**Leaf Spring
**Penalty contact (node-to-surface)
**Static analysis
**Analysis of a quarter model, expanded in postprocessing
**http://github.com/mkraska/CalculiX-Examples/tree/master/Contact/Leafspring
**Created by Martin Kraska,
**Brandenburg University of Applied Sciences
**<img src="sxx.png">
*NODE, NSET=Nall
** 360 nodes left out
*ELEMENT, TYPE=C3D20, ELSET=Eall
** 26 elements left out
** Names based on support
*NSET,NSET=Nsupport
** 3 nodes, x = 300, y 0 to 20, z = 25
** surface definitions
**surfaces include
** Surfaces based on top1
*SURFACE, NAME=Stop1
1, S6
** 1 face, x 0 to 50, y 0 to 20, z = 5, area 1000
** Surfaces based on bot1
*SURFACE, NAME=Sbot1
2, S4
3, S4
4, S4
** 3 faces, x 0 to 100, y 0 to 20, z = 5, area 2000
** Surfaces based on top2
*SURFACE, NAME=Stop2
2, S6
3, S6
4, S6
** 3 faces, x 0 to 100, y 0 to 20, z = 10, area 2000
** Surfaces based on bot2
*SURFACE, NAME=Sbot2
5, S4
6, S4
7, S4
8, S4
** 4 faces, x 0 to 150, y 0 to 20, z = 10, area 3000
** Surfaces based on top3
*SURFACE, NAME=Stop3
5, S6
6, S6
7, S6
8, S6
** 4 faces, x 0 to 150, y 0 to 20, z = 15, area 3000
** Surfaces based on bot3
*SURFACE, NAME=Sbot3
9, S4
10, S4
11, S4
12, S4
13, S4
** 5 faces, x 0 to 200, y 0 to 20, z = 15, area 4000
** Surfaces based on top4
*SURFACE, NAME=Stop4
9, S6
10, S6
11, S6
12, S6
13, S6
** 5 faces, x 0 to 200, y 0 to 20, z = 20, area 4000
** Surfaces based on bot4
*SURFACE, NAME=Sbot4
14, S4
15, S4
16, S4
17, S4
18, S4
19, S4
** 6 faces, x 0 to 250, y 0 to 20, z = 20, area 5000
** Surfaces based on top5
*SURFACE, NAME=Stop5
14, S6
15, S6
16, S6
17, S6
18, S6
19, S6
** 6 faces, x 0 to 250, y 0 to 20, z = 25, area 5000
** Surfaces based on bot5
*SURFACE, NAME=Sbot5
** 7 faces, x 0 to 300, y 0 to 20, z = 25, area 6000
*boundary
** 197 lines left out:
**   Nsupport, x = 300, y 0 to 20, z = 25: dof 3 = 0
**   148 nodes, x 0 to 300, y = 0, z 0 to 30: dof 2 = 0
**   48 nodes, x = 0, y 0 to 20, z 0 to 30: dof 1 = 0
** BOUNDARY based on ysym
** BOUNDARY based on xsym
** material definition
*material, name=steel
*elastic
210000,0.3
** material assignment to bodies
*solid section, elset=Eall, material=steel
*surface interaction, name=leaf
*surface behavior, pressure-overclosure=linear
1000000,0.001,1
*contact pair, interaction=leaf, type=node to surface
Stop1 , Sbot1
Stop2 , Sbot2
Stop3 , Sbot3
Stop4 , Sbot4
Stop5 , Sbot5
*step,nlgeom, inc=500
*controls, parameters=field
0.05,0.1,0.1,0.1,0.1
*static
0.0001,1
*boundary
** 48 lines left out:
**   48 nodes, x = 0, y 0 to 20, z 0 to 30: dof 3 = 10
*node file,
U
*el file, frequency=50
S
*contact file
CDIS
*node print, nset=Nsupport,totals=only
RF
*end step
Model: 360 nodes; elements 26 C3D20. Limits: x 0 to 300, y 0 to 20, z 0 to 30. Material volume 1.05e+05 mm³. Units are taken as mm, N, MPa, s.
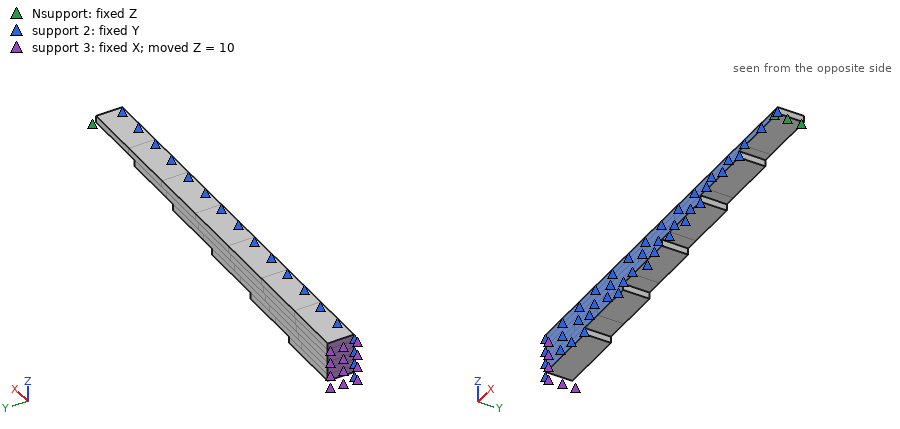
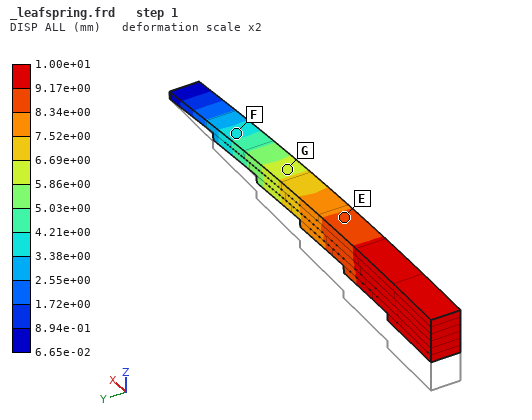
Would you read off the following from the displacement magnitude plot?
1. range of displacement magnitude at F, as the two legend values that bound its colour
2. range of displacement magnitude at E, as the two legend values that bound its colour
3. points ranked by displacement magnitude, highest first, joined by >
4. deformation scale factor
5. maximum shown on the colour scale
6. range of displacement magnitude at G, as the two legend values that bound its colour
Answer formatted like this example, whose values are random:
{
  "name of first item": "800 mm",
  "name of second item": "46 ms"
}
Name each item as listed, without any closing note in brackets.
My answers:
{
  "range of displacement magnitude at F, as the two legend values that bound its colour": "3.38e+00 to 4.21e+00 mm",
  "range of displacement magnitude at E, as the two legend values that bound its colour": "8.34e+00 to 9.17e+00 mm",
  "points ranked by displacement magnitude, highest first, joined by >": "E > G > F",
  "deformation scale factor": "2",
  "maximum shown on the colour scale": "1.00e+01 mm",
  "range of displacement magnitude at G, as the two legend values that bound its colour": "5.86e+00 to 6.69e+00 mm"
}
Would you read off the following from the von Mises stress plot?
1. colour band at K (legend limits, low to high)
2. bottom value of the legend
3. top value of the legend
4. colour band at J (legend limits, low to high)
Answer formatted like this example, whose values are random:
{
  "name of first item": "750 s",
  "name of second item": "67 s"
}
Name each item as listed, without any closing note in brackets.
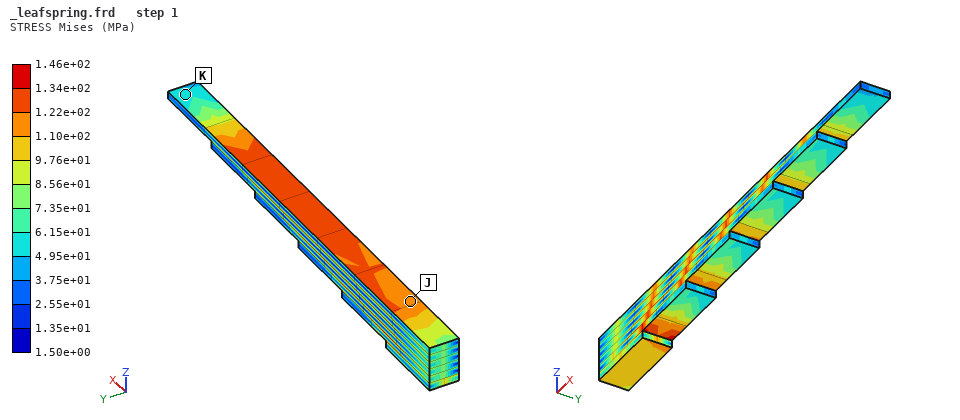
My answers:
{
  "colour band at K": "4.95e+01 to 6.15e+01 MPa",
  "bottom value of the legend": "1.50e+00 MPa",
  "top value of the legend": "1.46e+02 MPa",
  "colour band at J": "1.10e+02 to 1.22e+02 MPa"
}
